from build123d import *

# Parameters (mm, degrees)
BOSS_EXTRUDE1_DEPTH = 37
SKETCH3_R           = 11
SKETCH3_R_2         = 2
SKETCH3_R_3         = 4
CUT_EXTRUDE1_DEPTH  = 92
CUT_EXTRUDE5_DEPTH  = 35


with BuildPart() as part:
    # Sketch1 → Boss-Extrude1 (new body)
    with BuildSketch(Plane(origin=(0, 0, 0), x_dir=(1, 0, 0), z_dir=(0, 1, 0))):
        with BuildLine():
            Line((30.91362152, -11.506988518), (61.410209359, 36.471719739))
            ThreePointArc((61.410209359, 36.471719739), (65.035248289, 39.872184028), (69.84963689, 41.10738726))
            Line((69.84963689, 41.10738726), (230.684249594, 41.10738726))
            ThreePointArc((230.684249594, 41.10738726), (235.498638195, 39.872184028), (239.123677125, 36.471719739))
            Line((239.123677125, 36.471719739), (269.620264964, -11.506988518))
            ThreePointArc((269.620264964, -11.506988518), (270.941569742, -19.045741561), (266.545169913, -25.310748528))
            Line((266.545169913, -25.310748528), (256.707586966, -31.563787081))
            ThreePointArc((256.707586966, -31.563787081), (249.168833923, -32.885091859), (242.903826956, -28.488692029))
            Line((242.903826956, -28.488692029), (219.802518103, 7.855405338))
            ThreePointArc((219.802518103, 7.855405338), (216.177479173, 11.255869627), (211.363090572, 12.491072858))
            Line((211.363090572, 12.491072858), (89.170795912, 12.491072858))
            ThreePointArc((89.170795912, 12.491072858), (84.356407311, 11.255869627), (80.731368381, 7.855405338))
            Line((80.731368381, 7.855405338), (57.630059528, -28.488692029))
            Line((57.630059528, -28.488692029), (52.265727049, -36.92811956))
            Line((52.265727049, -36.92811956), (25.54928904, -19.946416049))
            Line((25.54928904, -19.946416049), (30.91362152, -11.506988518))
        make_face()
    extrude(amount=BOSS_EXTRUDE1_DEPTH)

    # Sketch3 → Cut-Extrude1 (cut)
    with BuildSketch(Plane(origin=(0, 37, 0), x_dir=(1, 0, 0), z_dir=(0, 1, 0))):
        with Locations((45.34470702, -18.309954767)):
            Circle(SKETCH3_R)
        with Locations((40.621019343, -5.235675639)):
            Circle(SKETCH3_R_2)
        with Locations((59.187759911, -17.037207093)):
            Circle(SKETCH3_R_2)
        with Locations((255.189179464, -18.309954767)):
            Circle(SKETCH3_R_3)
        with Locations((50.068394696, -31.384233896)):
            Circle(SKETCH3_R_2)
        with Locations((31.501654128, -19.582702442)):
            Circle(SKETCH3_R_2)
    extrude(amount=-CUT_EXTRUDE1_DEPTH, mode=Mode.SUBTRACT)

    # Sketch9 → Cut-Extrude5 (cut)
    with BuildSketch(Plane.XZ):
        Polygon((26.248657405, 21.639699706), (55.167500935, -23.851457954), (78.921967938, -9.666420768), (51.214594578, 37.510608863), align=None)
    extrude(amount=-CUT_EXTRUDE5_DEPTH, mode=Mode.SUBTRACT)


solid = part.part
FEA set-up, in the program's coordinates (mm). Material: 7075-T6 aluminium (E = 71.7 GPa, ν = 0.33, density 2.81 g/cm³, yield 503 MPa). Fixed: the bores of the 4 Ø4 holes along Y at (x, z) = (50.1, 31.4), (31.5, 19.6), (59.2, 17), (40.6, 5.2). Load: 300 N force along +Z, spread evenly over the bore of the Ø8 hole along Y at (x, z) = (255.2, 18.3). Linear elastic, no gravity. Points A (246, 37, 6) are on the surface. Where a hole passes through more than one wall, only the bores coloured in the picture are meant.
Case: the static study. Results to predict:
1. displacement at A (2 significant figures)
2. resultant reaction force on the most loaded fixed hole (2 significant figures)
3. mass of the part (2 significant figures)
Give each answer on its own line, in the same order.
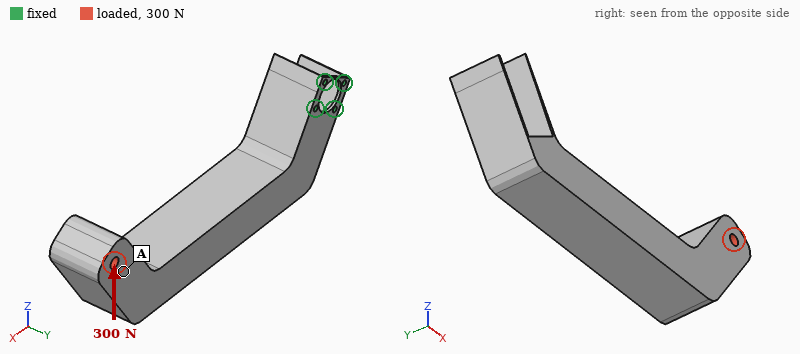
0.76 mm
2.1 kN
720 g
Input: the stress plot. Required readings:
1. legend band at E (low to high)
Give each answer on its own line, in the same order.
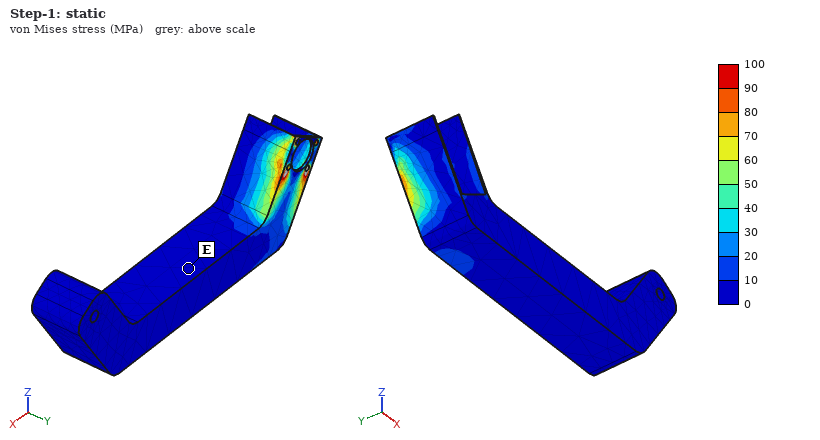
0 to 10 MPa
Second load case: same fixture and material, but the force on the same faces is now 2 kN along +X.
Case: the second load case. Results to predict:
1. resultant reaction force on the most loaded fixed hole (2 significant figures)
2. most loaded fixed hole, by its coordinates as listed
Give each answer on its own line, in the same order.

2.0 kN
(59.2, 17)
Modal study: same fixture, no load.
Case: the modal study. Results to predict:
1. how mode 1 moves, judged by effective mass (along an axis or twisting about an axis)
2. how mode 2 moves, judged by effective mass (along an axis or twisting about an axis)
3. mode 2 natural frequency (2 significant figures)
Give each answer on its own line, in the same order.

along Y
along Z
220 Hz
